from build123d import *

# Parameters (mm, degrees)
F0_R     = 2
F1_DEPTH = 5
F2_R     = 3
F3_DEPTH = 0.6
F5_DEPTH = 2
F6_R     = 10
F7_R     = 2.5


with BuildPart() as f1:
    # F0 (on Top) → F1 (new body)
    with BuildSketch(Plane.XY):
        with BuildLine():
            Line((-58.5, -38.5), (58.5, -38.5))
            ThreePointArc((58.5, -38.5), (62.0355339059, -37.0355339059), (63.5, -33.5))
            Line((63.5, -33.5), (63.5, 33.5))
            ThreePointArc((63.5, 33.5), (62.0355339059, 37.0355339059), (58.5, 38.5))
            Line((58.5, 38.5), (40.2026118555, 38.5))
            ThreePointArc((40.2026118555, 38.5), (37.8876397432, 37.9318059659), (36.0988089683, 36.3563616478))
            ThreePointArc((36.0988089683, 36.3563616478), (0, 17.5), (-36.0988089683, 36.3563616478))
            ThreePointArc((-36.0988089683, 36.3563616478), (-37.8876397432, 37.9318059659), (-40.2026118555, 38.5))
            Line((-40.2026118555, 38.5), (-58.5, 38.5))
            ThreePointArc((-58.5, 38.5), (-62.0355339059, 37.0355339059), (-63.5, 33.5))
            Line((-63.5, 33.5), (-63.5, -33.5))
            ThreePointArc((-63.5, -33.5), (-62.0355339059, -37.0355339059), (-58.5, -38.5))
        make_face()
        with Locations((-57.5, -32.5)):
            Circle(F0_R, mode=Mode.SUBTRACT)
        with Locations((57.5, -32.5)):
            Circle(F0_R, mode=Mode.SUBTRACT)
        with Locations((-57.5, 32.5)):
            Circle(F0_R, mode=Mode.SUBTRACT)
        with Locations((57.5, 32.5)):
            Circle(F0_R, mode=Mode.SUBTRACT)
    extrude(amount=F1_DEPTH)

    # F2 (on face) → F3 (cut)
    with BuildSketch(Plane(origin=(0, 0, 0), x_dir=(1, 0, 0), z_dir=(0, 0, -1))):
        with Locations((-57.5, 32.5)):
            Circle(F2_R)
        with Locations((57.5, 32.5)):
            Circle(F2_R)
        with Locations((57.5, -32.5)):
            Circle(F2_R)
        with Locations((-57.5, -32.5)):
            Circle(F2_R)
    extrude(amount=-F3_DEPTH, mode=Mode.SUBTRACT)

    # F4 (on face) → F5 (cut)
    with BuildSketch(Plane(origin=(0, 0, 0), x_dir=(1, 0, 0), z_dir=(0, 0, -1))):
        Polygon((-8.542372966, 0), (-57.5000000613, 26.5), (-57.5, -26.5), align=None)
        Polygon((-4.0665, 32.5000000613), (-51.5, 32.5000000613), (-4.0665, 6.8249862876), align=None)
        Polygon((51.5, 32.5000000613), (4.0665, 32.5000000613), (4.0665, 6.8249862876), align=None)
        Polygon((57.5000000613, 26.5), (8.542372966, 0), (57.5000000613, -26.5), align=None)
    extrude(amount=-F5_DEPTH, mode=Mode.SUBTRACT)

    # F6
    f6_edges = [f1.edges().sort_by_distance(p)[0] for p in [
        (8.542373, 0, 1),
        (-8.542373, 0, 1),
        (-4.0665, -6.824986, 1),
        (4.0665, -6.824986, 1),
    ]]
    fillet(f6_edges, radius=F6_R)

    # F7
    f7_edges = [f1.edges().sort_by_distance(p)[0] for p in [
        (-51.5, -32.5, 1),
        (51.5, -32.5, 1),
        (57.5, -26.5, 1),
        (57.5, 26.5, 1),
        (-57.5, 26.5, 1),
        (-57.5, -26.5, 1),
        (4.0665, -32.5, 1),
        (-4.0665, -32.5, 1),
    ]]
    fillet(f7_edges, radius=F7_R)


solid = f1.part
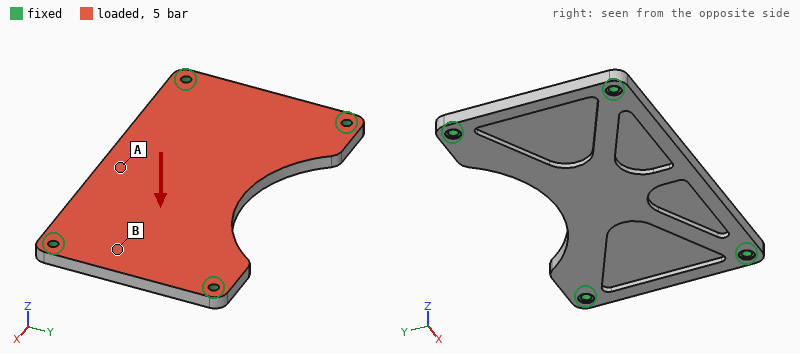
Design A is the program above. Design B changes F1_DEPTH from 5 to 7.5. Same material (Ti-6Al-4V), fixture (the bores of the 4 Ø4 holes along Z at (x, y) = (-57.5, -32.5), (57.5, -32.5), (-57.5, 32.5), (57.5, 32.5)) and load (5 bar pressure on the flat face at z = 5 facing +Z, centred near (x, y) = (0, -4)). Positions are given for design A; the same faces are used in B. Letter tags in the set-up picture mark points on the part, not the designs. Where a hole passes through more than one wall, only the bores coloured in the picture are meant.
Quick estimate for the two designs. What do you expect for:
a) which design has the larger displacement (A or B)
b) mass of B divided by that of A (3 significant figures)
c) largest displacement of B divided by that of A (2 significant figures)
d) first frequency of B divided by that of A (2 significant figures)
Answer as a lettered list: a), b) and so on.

a) A
b) 1.60
c) 0.30
d) 1.4
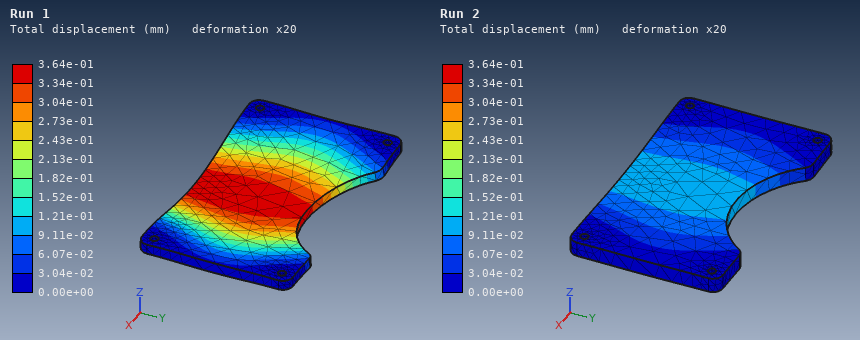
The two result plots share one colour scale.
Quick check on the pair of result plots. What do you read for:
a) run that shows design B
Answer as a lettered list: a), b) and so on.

a) Run 2
